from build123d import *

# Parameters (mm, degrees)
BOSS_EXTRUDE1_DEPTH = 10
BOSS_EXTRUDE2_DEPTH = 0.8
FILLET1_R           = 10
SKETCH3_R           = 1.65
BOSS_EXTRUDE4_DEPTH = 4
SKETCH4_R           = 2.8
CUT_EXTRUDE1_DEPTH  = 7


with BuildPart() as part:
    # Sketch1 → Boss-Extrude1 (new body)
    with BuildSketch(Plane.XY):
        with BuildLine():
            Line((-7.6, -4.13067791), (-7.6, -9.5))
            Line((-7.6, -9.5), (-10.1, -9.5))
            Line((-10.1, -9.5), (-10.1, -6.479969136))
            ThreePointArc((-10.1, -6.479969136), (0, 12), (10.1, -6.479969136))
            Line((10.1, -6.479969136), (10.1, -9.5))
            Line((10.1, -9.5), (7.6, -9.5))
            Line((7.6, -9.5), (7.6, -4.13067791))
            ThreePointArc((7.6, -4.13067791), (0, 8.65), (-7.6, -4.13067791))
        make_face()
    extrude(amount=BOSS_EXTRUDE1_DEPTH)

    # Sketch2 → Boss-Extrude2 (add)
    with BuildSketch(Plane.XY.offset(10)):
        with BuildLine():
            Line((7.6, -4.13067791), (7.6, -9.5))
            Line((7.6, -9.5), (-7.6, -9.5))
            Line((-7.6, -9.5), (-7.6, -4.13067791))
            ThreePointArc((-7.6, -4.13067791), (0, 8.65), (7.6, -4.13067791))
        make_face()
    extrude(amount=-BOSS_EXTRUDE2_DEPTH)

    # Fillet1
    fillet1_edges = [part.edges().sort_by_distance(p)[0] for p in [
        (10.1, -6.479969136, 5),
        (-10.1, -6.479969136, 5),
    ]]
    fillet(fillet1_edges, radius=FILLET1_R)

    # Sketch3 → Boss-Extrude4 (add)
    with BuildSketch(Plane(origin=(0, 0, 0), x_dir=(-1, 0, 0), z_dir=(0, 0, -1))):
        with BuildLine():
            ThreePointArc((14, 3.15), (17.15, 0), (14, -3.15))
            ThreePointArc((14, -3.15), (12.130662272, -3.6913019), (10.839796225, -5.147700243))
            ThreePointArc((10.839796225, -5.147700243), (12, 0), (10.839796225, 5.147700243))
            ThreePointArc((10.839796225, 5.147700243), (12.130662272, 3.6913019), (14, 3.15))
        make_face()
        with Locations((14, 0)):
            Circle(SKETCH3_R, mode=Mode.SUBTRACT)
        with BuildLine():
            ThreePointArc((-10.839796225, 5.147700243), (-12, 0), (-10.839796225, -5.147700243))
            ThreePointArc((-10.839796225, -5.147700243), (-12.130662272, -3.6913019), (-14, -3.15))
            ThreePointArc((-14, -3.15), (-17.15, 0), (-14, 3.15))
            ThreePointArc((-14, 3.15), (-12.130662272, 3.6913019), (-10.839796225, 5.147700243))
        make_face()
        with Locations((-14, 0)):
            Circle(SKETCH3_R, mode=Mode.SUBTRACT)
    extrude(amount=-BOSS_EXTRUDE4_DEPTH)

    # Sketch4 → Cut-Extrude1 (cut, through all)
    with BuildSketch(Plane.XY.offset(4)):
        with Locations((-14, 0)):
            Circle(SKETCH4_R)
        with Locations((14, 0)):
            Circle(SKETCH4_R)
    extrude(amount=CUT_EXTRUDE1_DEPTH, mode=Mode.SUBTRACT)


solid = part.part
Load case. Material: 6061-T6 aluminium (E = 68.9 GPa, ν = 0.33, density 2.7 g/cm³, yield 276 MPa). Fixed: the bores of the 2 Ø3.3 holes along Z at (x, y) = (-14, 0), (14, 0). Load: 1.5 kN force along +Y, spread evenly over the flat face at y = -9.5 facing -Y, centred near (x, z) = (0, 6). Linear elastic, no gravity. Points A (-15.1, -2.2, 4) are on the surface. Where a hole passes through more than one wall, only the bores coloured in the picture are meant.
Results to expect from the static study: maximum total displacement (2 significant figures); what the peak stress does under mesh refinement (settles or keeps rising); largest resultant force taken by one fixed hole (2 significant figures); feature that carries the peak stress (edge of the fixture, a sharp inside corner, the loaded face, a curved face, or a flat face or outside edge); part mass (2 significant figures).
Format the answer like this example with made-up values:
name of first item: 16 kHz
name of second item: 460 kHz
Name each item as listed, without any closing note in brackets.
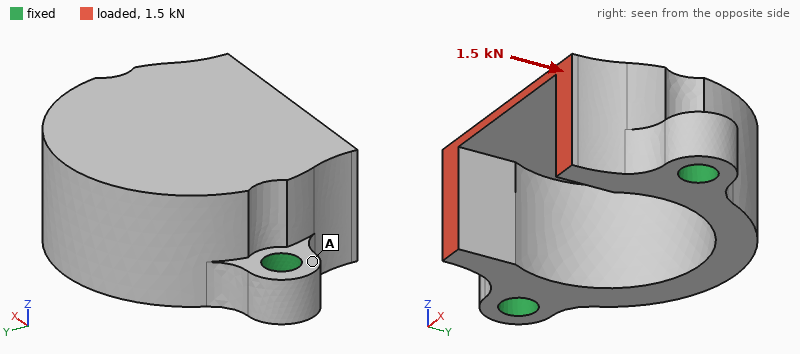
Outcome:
maximum total displacement: 48 µm
what the peak stress does under mesh refinement: keeps rising
largest resultant force taken by one fixed hole: 750 N
feature that carries the peak stress: edge of the fixture
part mass: 5.5 g
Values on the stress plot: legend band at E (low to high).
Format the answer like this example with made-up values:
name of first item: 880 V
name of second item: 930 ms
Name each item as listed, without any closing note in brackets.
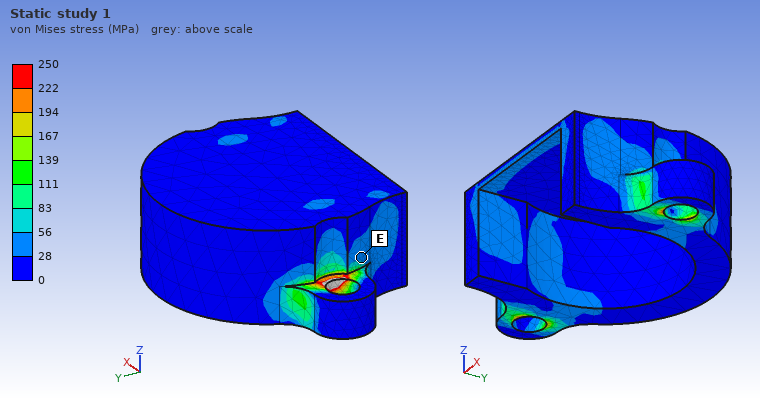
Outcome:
legend band at E: 28 to 56 MPa
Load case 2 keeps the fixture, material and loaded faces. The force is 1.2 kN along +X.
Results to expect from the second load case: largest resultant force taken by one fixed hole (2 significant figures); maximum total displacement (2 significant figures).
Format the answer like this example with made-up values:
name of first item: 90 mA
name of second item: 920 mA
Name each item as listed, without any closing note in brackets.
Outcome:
largest resultant force taken by one fixed hole: 680 N
maximum total displacement: 65 µm
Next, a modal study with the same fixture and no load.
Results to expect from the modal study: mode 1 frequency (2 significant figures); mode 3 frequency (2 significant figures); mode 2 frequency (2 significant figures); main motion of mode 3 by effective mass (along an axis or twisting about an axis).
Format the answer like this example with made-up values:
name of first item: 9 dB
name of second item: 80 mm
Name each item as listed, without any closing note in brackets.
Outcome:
mode 1 frequency: 12 kHz
mode 3 frequency: 19 kHz
mode 2 frequency: 17 kHz
main motion of mode 3 by effective mass: along X
